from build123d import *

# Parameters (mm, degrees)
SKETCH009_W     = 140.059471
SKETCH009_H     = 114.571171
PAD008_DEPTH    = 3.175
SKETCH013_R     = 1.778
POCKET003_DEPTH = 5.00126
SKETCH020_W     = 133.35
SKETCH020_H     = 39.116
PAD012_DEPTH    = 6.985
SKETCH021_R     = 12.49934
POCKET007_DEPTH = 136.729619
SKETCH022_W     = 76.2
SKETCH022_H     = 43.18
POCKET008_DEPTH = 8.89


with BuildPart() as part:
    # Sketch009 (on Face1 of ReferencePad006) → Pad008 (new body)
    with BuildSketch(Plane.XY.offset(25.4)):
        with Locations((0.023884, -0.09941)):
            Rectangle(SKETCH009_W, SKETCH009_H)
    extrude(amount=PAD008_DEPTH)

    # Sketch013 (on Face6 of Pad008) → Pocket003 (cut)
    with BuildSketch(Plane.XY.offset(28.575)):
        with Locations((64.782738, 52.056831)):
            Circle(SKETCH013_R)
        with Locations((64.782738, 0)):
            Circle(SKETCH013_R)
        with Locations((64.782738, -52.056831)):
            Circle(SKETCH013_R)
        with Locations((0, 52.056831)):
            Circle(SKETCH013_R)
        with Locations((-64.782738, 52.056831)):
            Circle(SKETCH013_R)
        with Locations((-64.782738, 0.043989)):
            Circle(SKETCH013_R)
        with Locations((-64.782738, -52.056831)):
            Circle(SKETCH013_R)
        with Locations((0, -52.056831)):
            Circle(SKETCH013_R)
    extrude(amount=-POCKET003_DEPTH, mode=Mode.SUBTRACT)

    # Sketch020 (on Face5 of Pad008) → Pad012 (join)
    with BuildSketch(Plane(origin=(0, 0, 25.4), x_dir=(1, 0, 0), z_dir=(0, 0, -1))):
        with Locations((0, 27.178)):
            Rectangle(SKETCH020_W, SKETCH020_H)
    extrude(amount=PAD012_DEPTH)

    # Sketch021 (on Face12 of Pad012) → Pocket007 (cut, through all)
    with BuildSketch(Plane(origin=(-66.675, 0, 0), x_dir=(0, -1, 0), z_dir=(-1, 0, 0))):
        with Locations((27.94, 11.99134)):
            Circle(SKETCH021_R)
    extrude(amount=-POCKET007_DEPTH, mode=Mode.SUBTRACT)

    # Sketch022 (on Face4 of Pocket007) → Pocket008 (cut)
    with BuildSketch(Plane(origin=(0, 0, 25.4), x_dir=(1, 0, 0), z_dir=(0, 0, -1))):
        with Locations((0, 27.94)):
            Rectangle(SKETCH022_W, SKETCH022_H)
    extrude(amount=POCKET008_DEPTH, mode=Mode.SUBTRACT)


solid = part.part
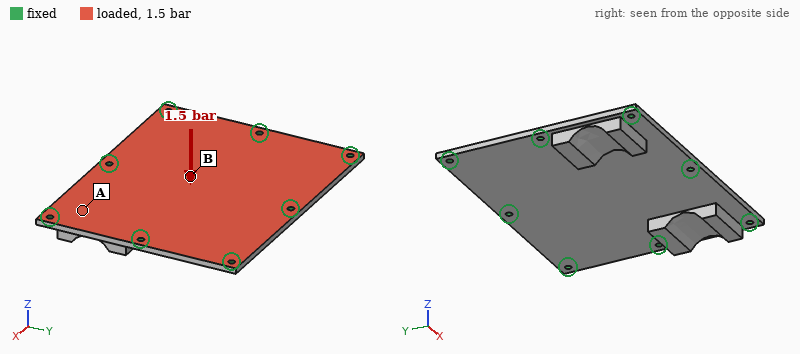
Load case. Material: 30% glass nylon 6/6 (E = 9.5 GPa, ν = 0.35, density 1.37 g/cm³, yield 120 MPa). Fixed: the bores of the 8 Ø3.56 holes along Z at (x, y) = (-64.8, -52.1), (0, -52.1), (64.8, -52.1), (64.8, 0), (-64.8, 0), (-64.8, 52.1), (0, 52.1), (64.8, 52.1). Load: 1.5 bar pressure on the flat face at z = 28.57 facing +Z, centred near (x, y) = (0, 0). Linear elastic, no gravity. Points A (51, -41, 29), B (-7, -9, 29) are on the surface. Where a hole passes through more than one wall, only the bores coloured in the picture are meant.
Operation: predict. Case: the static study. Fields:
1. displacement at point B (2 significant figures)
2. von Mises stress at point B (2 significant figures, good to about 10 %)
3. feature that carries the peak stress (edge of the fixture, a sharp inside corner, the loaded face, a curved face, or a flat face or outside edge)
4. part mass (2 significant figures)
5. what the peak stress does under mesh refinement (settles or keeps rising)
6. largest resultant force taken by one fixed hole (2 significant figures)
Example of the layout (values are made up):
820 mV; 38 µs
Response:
1.4 mm; 26 MPa; edge of the fixture; 84 g; keeps rising; 520 N
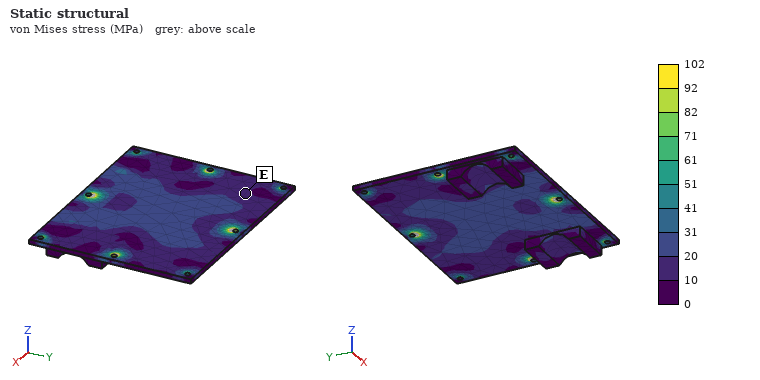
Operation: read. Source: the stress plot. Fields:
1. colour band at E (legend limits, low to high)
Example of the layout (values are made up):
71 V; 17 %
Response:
10 to 20 MPa
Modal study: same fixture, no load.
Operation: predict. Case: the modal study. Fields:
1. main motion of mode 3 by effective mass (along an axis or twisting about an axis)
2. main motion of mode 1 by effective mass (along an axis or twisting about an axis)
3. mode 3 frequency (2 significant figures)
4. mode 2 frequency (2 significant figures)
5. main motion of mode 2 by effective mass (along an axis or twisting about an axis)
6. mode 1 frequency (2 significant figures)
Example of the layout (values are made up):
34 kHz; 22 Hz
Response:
twisting about X; along Z; 1700 Hz; 1400 Hz; twisting about Y; 950 Hz
